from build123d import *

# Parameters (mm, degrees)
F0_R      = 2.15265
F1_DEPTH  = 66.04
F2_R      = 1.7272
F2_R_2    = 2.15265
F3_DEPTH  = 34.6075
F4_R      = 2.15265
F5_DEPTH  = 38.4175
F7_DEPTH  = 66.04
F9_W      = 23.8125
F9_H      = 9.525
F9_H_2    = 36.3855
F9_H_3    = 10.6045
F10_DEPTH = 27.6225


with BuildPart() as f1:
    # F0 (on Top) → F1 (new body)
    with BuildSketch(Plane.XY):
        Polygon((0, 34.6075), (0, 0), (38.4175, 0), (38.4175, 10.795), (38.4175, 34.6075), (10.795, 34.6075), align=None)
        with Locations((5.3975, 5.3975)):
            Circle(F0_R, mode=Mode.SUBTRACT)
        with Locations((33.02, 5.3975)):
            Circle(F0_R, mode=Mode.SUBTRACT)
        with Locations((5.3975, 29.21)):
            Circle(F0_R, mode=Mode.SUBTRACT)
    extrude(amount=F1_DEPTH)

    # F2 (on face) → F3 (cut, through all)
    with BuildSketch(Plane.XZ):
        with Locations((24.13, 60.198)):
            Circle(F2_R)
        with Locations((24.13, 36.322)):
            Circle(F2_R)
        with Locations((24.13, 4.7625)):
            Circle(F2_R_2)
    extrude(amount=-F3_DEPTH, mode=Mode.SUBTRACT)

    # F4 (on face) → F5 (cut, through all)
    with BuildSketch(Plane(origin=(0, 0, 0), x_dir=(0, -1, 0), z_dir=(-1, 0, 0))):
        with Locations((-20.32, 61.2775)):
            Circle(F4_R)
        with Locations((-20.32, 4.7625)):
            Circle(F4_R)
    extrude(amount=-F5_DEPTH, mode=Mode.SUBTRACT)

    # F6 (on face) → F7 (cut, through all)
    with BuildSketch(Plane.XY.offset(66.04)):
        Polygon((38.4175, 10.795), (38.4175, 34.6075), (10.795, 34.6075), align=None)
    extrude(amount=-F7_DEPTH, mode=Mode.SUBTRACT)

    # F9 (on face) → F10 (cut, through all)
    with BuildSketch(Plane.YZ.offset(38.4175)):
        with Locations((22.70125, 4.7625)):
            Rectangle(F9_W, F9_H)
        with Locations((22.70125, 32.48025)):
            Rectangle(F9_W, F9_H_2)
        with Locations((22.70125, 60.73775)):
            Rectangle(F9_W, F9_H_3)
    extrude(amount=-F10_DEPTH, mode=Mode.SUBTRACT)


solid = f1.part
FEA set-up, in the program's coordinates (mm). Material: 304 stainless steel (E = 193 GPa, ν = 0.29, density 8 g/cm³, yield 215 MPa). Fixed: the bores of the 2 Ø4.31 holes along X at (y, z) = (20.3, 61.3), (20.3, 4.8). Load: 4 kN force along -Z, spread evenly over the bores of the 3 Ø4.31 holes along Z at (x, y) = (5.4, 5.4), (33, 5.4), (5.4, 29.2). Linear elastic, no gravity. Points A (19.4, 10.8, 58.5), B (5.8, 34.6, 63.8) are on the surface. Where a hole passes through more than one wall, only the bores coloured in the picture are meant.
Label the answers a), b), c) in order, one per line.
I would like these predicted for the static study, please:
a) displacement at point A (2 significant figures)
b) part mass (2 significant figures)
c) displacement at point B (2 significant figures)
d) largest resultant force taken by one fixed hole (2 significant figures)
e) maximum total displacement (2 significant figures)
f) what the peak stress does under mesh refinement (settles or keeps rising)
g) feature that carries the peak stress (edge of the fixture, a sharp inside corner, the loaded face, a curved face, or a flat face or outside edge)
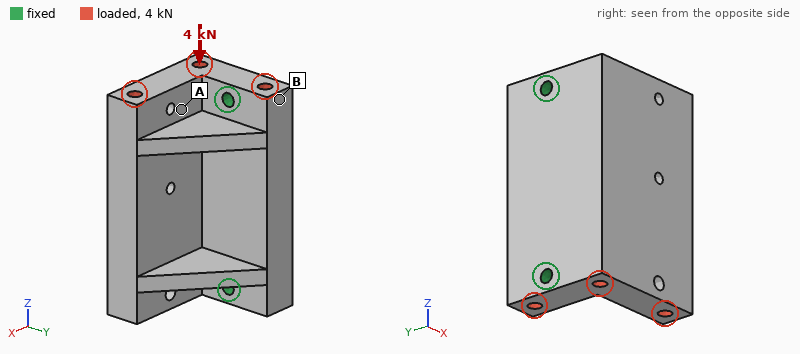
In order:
a) 2.4 µm
b) 350 g
c) 0.83 µm
d) 2.2 kN
e) 4.4 µm
f) keeps rising
g) edge of the fixture
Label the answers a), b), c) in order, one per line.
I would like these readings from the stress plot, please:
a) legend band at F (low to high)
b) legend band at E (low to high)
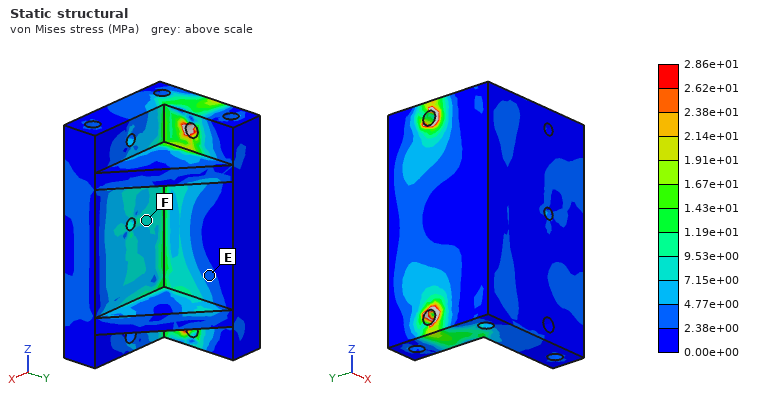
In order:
a) 7.15e+00 to 9.53e+00 MPa
b) 2.38e+00 to 4.77e+00 MPa
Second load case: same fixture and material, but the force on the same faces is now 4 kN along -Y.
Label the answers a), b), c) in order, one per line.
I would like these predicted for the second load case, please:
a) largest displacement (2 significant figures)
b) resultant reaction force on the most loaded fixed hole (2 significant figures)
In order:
a) 18 µm
b) 2.0 kN
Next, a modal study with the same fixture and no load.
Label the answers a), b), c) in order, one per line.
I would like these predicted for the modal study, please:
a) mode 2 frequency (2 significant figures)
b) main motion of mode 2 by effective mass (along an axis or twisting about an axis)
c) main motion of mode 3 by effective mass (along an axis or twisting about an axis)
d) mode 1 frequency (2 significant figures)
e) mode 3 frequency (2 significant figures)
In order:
a) 8400 Hz
b) along Z
c) along X
d) 4600 Hz
e) 12 kHz
